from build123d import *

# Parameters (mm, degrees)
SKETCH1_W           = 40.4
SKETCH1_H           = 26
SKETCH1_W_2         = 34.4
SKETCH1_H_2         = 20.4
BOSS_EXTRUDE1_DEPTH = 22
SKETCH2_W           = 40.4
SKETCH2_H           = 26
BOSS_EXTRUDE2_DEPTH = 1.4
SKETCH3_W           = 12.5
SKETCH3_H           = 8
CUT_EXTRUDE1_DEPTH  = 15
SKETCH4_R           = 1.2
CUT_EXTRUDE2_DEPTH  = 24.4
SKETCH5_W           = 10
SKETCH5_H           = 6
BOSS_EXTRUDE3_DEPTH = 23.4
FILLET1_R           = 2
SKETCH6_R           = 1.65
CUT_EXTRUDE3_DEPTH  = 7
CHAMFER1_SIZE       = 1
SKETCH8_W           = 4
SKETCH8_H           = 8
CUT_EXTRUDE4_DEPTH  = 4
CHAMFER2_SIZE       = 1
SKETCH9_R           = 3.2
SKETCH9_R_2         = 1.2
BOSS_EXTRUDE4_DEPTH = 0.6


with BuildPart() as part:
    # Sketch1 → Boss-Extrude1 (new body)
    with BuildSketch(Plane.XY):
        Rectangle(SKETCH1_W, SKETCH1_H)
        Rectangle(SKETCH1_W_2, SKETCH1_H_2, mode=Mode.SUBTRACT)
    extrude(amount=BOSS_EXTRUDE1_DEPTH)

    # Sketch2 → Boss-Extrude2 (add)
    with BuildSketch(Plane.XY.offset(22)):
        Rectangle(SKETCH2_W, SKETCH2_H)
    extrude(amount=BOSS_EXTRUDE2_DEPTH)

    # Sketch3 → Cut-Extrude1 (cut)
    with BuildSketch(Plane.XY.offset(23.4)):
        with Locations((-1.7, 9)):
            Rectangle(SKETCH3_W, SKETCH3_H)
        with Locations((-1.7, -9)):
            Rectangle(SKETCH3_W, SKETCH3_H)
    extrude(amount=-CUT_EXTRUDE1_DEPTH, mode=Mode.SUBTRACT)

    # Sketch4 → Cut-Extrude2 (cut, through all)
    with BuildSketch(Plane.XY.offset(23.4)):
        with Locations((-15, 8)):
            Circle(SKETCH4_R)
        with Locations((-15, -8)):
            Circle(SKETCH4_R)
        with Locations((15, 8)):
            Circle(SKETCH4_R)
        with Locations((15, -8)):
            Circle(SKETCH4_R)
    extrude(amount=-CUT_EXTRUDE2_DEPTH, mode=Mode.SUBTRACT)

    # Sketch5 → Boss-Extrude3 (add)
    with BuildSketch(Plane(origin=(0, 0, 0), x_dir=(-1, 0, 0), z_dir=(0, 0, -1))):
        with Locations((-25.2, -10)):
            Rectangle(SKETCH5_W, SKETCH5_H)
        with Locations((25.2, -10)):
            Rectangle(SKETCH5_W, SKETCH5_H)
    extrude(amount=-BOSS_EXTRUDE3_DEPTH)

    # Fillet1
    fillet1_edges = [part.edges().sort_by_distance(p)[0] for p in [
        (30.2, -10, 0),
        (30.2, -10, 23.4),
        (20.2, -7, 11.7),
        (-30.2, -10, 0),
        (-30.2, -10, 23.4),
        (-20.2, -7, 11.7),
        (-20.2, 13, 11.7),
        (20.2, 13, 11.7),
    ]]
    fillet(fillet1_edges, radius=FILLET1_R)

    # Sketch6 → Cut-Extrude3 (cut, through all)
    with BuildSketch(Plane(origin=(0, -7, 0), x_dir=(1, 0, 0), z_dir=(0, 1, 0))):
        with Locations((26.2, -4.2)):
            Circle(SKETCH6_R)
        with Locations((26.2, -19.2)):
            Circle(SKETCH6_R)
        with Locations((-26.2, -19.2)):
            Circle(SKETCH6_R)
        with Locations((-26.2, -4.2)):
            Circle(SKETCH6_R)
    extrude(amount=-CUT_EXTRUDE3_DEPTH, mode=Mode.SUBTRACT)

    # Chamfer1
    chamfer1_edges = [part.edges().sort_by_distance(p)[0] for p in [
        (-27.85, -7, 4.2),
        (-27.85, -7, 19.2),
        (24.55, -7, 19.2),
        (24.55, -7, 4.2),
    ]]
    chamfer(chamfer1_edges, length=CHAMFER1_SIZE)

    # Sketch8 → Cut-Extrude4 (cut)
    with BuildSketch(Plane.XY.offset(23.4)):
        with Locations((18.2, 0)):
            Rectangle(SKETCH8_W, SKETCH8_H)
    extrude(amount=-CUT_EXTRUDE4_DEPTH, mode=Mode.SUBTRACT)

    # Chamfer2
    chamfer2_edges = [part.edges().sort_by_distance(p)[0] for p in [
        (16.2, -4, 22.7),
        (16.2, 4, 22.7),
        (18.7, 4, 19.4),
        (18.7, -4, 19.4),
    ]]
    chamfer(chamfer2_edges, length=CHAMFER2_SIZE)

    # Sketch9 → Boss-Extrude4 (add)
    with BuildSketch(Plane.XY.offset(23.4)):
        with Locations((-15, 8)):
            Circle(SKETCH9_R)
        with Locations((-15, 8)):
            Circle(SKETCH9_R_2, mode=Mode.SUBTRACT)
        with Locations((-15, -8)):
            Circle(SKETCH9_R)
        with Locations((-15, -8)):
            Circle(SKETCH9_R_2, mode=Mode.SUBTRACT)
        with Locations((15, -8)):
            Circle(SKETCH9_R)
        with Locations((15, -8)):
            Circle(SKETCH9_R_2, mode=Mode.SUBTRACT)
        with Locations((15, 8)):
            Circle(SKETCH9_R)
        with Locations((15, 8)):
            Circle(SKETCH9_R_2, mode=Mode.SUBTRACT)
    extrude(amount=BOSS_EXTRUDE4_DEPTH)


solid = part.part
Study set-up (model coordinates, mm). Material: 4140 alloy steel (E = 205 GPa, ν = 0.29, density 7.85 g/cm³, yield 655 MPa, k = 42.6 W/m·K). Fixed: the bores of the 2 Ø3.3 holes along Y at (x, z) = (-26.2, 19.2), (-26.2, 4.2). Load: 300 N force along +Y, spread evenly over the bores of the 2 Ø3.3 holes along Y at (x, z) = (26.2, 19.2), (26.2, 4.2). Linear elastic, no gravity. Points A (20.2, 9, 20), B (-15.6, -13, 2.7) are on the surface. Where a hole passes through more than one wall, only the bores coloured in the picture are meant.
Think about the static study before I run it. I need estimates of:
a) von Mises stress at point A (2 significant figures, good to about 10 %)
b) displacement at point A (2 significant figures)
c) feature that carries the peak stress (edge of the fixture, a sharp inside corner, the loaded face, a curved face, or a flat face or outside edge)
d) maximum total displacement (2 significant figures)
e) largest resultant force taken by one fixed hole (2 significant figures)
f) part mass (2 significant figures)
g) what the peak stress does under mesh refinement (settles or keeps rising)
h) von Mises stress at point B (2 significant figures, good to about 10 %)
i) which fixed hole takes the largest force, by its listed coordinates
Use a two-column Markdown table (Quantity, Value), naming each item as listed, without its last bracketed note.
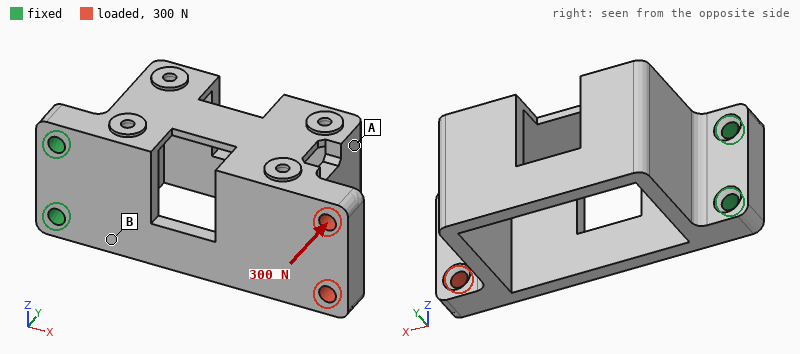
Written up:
| Quantity | Value |
|---|---|
| von Mises stress at point A | 29 MPa |
| displacement at point A | 0.19 mm |
| feature that carries the peak stress | edge of the fixture |
| maximum total displacement | 0.25 mm |
| largest resultant force taken by one fixed hole | 170 N |
| part mass | 82 g |
| what the peak stress does under mesh refinement | keeps rising |
| von Mises stress at point B | 94 MPa |
| which fixed hole takes the largest force, by its listed coordinates | (-26.2, 4.2) |
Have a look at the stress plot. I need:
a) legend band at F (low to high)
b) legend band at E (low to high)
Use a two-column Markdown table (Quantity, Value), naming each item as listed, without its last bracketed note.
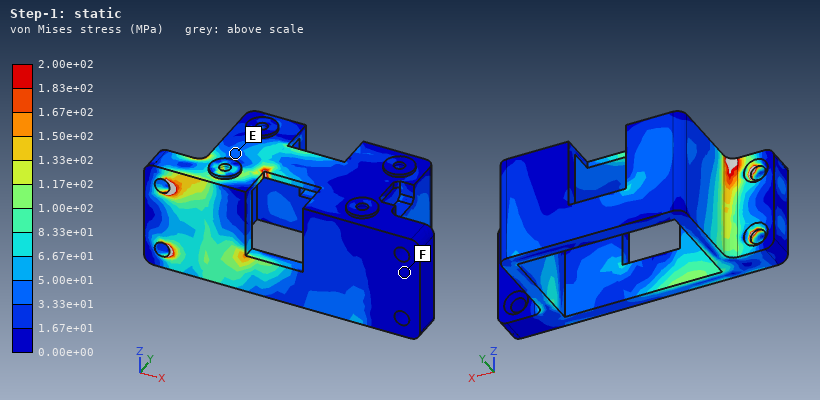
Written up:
| Quantity | Value |
|---|---|
| legend band at F | 0.00e+00 to 1.67e+01 MPa |
| legend band at E | 3.33e+01 to 5.00e+01 MPa |
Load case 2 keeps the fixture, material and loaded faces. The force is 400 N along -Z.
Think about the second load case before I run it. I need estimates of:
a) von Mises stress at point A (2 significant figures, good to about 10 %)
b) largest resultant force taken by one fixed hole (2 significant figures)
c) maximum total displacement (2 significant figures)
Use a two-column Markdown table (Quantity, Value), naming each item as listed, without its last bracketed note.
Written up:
| Quantity | Value |
|---|---|
| von Mises stress at point A | 9.7 MPa |
| largest resultant force taken by one fixed hole | 1.3 kN |
| maximum total displacement | 93 µm |
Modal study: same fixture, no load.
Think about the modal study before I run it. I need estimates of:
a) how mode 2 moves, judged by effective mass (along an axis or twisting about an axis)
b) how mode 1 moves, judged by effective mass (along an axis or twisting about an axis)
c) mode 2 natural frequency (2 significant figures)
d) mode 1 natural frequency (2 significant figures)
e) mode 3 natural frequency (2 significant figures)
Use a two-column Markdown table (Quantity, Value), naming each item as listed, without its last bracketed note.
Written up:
| Quantity | Value |
|---|---|
| how mode 2 moves, judged by effective mass | along Z |
| how mode 1 moves, judged by effective mass | along Y |
| mode 2 natural frequency | 2200 Hz |
| mode 1 natural frequency | 1100 Hz |
| mode 3 natural frequency | 3500 Hz |
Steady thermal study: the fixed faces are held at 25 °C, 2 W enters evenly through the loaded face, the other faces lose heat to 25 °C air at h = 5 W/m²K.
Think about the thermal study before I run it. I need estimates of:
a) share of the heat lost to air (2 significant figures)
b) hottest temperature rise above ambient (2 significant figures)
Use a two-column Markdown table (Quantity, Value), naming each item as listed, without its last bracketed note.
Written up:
| Quantity | Value |
|---|---|
| share of the heat lost to air | 24 % |
| hottest temperature rise above ambient | 26 K |
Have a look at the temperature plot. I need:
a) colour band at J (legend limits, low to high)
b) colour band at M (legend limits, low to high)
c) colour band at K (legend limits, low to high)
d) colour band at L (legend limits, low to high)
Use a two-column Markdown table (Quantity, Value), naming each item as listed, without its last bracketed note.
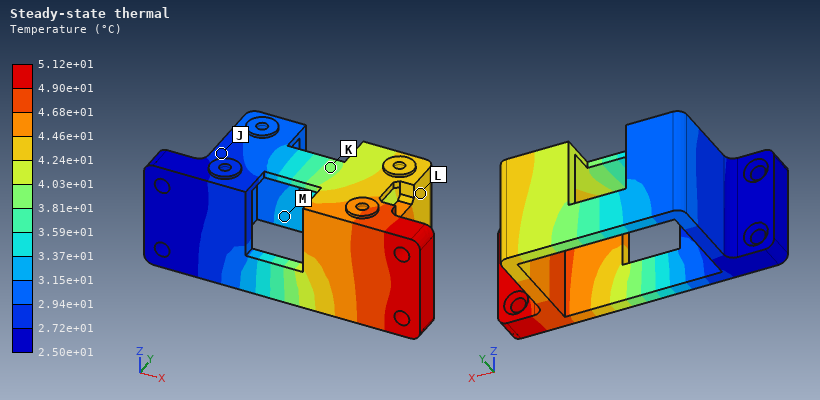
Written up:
| Quantity | Value |
|---|---|
| colour band at J | 2.72e+01 to 2.94e+01 °C |
| colour band at M | 3.15e+01 to 3.37e+01 °C |
| colour band at K | 3.81e+01 to 4.03e+01 °C |
| colour band at L | 4.24e+01 to 4.46e+01 °C |
